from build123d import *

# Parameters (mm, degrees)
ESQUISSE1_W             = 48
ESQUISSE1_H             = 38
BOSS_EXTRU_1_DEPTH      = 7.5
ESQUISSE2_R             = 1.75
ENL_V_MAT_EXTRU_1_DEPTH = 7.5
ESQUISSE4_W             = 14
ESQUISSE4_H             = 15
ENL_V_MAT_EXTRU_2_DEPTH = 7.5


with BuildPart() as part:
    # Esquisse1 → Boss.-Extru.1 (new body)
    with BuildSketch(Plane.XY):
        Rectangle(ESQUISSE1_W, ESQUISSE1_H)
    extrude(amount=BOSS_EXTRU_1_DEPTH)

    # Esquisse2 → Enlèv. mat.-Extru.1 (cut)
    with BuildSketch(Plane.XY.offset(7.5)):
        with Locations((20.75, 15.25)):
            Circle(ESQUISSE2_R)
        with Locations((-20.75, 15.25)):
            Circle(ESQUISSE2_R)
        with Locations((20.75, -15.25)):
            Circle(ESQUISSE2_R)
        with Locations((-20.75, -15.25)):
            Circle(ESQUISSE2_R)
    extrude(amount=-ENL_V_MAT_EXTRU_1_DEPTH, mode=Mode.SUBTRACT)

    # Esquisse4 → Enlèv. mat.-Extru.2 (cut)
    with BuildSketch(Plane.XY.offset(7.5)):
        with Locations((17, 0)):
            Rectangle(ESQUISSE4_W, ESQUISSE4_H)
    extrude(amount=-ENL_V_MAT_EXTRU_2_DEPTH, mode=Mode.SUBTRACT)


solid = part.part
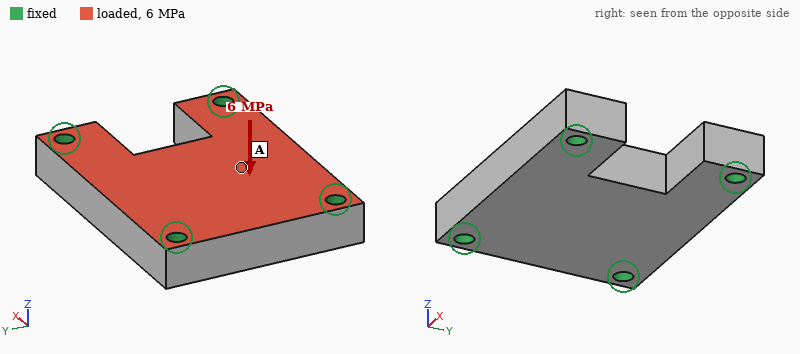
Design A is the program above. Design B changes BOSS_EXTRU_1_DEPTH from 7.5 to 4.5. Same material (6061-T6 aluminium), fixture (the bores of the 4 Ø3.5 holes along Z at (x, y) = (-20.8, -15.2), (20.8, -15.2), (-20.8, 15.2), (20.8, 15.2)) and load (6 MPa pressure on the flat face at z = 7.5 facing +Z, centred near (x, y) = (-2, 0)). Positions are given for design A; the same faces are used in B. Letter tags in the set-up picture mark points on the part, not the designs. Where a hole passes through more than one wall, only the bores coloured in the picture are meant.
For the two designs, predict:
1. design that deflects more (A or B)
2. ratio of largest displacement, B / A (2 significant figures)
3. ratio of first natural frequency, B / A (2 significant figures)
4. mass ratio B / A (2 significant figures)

B
3.6
0.69
0.60
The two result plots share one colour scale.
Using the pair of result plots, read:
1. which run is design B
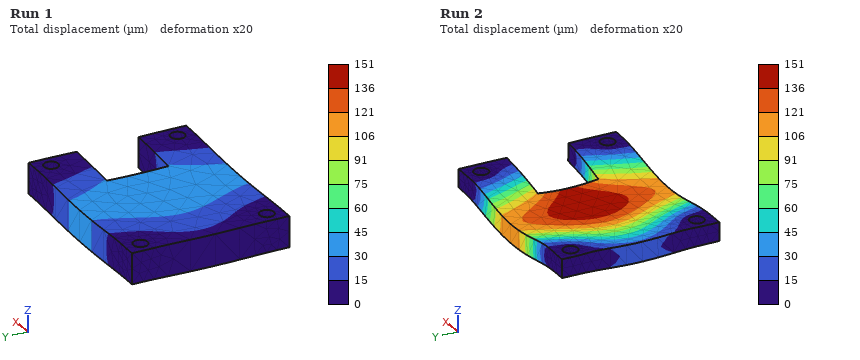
Run 2
